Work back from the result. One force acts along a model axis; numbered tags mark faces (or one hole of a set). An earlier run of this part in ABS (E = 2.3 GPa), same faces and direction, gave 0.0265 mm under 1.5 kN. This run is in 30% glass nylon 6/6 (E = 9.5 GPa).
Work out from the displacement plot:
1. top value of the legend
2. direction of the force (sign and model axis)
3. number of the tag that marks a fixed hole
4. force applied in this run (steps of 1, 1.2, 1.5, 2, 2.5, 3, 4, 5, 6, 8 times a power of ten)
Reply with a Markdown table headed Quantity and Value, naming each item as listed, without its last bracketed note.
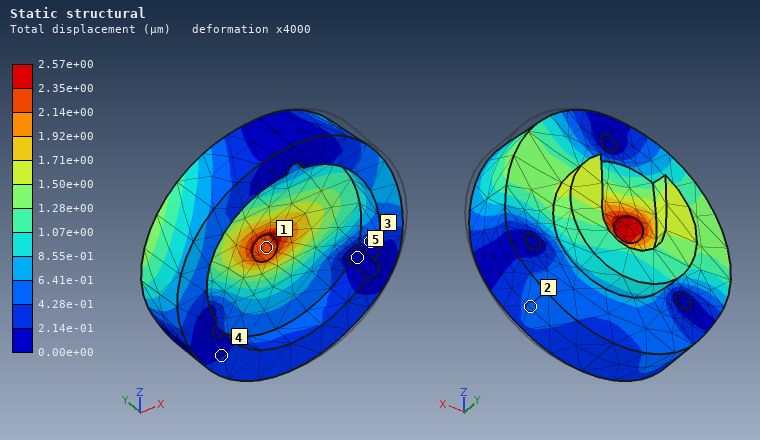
| Quantity | Value |
|---|---|
| top value of the legend | 2.57e+00 µm |
| direction of the force | -X |
| number of the tag that marks a fixed hole | 5 |
| force applied in this run | 600 N |
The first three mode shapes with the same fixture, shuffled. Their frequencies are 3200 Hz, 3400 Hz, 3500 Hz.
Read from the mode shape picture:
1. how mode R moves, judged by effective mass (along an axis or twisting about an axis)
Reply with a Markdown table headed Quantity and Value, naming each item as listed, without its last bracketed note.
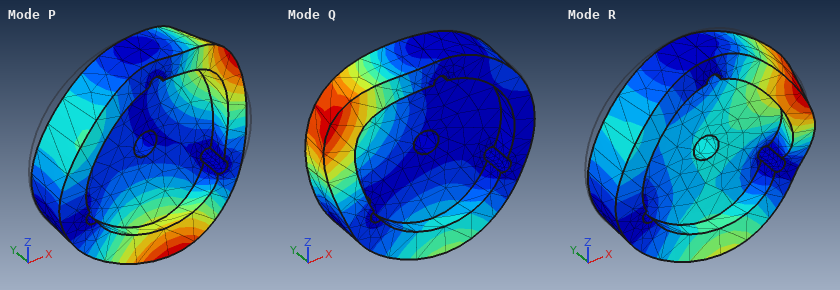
| Quantity | Value |
|---|---|
| how mode R moves, judged by effective mass | along Y |
